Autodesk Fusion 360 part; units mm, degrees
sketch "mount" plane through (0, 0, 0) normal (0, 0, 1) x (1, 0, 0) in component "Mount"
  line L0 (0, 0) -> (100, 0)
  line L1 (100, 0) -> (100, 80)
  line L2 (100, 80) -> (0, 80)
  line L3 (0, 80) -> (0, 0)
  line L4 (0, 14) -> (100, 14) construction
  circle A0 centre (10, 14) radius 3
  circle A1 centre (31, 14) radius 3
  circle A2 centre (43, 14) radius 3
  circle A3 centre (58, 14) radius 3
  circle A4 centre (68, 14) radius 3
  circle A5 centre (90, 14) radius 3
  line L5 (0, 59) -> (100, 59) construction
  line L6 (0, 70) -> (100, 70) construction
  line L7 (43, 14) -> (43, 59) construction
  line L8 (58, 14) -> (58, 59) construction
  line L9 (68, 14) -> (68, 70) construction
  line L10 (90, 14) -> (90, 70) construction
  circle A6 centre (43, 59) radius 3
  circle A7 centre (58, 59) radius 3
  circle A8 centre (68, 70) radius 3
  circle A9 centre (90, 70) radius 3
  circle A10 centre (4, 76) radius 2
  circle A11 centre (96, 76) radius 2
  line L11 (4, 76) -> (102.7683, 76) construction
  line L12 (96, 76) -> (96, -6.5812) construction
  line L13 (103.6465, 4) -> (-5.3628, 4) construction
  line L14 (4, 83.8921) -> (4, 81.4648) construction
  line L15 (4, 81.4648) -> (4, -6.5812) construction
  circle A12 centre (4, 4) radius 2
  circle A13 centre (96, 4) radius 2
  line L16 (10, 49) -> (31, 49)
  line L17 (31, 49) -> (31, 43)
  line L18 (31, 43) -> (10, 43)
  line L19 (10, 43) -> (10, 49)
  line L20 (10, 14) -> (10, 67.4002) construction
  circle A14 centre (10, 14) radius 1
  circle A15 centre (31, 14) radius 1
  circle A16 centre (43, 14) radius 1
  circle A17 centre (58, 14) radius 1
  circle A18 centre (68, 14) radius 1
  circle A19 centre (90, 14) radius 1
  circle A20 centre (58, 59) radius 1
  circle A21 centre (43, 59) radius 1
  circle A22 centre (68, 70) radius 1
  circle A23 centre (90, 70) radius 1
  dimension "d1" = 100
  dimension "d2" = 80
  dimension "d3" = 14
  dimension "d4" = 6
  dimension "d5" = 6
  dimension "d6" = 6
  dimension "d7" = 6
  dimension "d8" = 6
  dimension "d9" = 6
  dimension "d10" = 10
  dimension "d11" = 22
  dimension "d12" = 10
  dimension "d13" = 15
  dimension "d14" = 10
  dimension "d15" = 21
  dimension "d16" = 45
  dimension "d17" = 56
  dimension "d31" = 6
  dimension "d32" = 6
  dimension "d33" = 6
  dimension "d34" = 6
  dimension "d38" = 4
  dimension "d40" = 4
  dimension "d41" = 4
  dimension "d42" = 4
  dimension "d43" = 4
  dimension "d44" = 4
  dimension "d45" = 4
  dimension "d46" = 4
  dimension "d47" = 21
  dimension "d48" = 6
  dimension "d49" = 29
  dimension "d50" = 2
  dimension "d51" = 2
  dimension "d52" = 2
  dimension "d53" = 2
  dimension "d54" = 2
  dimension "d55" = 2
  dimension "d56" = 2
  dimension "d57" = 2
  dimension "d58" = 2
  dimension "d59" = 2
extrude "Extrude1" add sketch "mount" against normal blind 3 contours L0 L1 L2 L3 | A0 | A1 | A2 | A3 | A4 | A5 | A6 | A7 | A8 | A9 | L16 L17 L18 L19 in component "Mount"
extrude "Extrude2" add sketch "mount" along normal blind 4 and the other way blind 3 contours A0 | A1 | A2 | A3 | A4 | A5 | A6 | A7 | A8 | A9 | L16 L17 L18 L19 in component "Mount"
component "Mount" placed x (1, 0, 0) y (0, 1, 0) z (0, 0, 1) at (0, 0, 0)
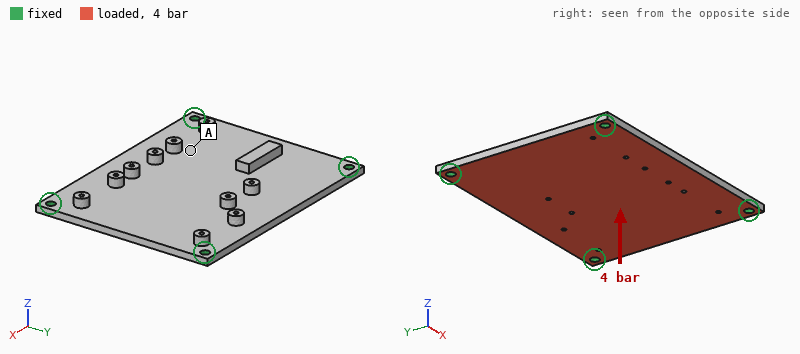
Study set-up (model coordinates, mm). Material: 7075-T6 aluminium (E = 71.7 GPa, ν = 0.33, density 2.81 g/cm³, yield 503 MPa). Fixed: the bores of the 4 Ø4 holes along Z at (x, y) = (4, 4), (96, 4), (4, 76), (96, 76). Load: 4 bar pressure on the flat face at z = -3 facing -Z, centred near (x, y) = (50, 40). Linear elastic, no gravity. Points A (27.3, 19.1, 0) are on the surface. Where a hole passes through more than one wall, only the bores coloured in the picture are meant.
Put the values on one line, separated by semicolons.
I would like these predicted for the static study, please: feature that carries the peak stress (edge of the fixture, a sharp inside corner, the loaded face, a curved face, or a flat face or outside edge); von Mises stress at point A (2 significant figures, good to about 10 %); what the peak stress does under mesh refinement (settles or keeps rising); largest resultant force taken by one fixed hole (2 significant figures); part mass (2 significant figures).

edge of the fixture; 58 MPa; keeps rising; 790 N; 71 g
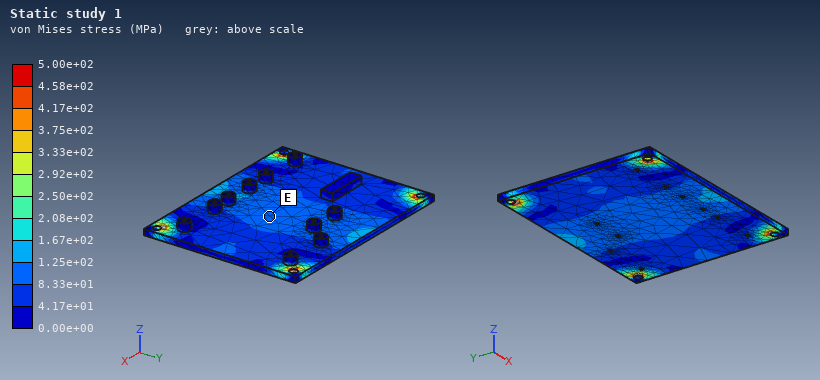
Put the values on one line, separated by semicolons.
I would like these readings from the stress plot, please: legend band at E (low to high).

8.33e+01 to 1.25e+02 MPa
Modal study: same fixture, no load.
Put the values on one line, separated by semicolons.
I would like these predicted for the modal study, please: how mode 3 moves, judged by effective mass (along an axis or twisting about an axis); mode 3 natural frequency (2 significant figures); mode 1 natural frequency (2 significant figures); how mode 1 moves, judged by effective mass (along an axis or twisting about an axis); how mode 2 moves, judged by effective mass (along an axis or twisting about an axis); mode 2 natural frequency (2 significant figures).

twisting about Y; 2900 Hz; 1300 Hz; along Z; twisting about X; 2200 Hz
